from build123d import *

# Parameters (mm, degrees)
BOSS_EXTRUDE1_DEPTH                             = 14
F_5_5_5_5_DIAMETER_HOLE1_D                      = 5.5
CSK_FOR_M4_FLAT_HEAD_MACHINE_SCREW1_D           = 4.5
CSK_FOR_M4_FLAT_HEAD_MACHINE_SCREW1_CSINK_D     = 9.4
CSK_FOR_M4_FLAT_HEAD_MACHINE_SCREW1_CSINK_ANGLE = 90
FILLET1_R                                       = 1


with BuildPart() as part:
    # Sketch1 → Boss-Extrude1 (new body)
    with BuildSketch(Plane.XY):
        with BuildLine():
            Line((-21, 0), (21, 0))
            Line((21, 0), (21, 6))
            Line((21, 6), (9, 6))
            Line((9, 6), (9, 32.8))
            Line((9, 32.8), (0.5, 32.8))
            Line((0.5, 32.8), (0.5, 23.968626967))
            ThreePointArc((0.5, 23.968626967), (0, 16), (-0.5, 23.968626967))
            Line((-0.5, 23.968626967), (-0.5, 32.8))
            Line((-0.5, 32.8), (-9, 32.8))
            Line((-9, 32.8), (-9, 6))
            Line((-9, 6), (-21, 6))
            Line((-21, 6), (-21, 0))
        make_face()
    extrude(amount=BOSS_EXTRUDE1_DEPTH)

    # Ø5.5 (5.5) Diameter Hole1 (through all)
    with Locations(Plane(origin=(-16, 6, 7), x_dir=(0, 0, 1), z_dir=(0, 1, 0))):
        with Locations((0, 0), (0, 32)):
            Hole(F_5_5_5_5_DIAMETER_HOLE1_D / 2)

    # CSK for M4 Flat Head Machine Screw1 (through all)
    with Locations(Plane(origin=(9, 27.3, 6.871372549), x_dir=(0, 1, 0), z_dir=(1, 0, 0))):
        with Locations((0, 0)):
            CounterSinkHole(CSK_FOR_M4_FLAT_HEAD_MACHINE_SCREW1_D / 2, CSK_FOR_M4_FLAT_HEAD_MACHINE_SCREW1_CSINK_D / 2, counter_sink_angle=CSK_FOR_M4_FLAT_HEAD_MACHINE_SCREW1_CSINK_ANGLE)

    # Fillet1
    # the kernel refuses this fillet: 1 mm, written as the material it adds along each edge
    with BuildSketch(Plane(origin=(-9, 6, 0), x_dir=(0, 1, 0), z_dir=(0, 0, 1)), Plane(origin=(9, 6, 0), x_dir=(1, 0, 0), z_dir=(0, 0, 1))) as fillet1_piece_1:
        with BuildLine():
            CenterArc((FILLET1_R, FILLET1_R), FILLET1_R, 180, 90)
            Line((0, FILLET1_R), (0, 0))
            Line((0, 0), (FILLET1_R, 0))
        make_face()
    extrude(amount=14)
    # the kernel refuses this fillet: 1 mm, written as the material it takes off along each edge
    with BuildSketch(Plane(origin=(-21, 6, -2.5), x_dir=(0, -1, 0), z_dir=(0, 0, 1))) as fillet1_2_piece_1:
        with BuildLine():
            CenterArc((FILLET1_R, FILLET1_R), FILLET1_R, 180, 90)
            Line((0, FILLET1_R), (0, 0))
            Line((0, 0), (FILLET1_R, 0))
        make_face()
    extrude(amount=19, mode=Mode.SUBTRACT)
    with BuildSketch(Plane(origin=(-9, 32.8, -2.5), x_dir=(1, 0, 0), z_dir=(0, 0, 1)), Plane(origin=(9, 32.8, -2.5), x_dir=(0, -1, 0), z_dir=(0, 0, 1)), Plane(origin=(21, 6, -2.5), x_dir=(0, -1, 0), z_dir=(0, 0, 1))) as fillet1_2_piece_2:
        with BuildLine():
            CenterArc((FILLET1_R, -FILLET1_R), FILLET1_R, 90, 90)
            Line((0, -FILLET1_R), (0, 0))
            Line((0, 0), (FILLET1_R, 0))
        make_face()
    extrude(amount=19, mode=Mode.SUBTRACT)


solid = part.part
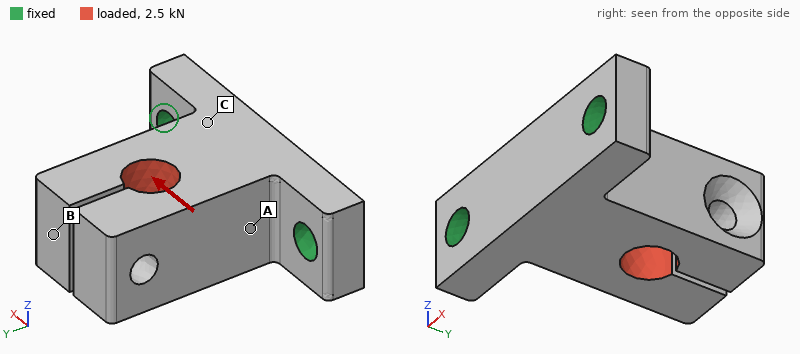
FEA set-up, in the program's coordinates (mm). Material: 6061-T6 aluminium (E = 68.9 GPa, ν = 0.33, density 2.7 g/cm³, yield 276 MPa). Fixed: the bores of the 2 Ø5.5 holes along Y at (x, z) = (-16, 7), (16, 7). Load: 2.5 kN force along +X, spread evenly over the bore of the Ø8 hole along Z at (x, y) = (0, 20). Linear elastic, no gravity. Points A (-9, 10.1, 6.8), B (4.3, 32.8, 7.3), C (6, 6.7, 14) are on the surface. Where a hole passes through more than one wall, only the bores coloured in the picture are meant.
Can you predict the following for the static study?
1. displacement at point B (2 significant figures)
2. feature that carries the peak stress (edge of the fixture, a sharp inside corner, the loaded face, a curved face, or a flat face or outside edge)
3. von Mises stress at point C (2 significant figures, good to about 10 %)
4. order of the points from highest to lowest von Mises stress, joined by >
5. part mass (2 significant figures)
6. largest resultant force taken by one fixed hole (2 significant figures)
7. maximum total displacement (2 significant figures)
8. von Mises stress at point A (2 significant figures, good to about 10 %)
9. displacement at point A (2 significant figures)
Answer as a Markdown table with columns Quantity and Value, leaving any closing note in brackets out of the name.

| Quantity | Value |
|---|---|
| displacement at point B | 70 µm |
| feature that carries the peak stress | a curved face |
| von Mises stress at point C | 24 MPa |
| order of the points from highest to lowest von Mises stress, joined by > | A > C > B |
| part mass | 24 g |
| largest resultant force taken by one fixed hole | 2.1 kN |
| maximum total displacement | 71 µm |
| von Mises stress at point A | 43 MPa |
| displacement at point A | 15 µm |
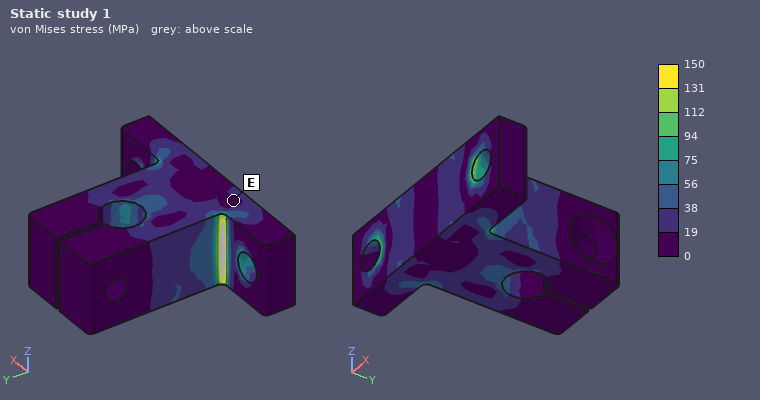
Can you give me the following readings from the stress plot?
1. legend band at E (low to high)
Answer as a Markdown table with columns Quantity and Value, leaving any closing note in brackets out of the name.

| Quantity | Value |
|---|---|
| legend band at E | 0 to 19 MPa |
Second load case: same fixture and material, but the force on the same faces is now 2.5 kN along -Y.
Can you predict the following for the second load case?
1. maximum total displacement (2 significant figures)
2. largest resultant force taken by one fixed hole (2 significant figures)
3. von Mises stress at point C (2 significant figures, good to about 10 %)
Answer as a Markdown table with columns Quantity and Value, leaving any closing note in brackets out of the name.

| Quantity | Value |
|---|---|
| maximum total displacement | 33 µm |
| largest resultant force taken by one fixed hole | 1.4 kN |
| von Mises stress at point C | 19 MPa |
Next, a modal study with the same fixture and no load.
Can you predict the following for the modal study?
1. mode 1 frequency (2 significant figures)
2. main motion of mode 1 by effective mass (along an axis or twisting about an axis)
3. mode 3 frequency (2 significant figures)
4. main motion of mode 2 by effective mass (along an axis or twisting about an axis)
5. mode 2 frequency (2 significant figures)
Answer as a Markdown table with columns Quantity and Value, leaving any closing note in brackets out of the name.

| Quantity | Value |
|---|---|
| mode 1 frequency | 5200 Hz |
| main motion of mode 1 by effective mass | along Z |
| mode 3 frequency | 10 kHz |
| main motion of mode 2 by effective mass | along X |
| mode 2 frequency | 8400 Hz |
